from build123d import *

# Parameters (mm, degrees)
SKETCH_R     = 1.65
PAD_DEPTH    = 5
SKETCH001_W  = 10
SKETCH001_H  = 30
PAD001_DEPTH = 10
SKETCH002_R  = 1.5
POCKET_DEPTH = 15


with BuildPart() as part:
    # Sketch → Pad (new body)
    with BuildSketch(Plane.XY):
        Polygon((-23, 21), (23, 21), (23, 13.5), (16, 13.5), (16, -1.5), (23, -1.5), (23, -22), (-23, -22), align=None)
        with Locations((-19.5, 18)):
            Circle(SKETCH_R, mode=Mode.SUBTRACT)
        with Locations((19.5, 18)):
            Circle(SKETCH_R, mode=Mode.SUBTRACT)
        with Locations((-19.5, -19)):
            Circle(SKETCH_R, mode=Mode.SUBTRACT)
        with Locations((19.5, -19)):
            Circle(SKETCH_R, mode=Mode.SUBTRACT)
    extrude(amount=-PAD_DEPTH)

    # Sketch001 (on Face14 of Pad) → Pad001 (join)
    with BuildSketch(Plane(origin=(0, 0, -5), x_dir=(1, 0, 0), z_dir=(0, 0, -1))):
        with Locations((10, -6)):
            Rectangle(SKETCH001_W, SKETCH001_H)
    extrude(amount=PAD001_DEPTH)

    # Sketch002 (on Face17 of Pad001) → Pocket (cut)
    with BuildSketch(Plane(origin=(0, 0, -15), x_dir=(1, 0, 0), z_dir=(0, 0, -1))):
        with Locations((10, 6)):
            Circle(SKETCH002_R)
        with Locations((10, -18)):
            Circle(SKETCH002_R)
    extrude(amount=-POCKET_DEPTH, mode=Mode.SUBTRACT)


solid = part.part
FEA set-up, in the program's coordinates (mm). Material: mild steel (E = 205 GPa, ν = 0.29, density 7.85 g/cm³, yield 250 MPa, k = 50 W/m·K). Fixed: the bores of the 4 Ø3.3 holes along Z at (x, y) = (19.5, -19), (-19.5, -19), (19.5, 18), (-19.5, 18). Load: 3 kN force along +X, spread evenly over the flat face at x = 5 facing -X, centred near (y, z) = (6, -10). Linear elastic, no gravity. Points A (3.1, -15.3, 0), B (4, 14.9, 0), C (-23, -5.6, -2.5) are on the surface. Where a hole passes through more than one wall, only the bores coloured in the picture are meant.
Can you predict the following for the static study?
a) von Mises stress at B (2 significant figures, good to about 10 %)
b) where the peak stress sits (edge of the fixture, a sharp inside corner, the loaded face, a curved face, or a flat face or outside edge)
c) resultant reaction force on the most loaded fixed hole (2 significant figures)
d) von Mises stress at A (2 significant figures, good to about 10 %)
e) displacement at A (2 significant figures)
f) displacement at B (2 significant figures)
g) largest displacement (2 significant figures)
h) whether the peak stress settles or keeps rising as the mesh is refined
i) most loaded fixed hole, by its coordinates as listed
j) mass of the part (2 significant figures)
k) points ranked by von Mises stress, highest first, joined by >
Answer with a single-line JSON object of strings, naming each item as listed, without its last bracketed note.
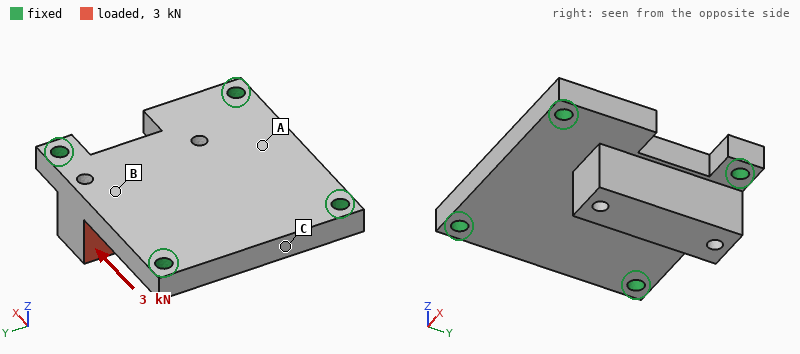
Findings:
{"von Mises stress at B": "57 MPa", "where the peak stress sits": "edge of the fixture", "resultant reaction force on the most loaded fixed hole": "1.3 kN", "von Mises stress at A": "24 MPa", "displacement at A": "4.2 µm", "displacement at B": "8.8 µm", "largest displacement": "17 µm", "whether the peak stress settles or keeps rising as the mesh is refined": "keeps rising", "most loaded fixed hole, by its coordinates as listed": "(19.5, 18)", "mass of the part": "94 g", "points ranked by von Mises stress, highest first, joined by >": "B > A > C"}
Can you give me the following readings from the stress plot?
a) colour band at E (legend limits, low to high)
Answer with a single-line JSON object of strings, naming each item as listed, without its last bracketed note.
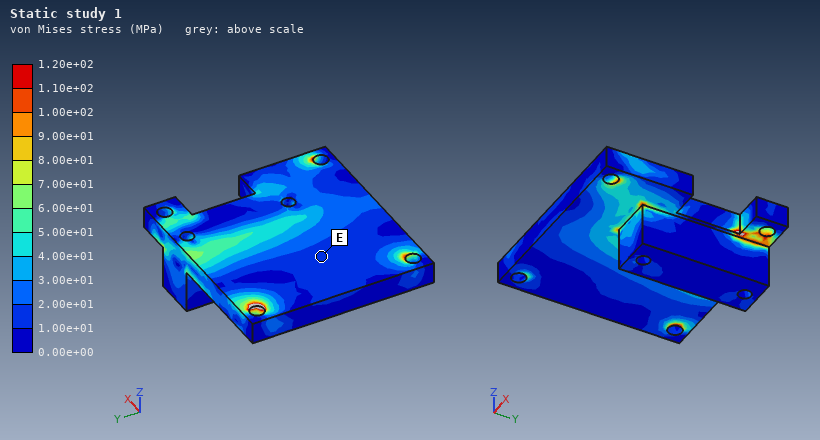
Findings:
{"colour band at E": "1.00e+01 to 2.00e+01 MPa"}
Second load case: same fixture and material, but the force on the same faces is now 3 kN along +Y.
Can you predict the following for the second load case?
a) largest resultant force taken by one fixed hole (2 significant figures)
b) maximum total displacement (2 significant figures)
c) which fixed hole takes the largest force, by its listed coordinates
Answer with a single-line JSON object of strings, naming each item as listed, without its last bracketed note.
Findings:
{"largest resultant force taken by one fixed hole": "1.4 kN", "maximum total displacement": "9.1 µm", "which fixed hole takes the largest force, by its listed coordinates": "(19.5, -19)"}
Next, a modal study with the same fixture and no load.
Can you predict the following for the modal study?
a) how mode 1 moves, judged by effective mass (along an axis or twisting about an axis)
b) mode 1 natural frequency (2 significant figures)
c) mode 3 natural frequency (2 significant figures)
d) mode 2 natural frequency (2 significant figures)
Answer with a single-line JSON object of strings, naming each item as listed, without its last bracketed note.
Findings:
{"how mode 1 moves, judged by effective mass": "along Z", "mode 1 natural frequency": "9600 Hz", "mode 3 natural frequency": "19 kHz", "mode 2 natural frequency": "15 kHz"}
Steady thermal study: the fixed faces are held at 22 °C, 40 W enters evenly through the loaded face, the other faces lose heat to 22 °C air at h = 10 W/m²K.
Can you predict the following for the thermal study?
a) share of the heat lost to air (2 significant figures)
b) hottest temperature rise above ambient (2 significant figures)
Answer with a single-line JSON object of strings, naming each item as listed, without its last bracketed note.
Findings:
{"share of the heat lost to air": "4.1 %", "hottest temperature rise above ambient": "74 K"}
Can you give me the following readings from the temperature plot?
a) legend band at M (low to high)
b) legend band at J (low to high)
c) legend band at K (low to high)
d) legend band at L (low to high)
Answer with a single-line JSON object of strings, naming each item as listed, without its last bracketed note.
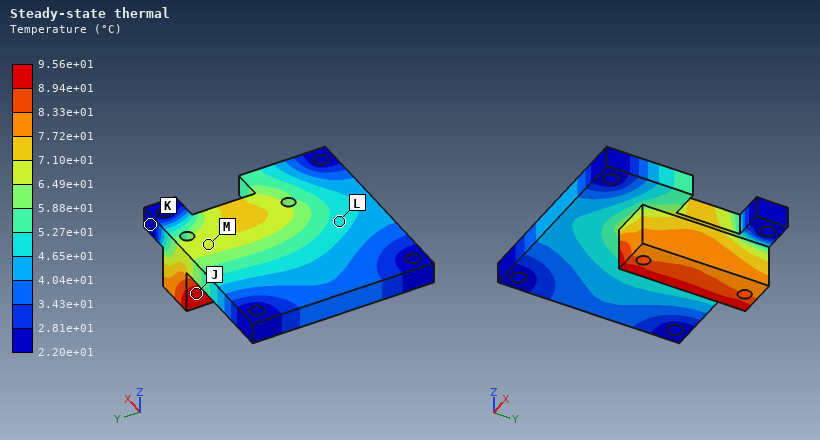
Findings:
{"legend band at M": "6.49e+01 to 7.10e+01 °C", "legend band at J": "8.94e+01 to 9.56e+01 °C", "legend band at K": "2.20e+01 to 2.81e+01 °C", "legend band at L": "4.65e+01 to 5.27e+01 °C"}
